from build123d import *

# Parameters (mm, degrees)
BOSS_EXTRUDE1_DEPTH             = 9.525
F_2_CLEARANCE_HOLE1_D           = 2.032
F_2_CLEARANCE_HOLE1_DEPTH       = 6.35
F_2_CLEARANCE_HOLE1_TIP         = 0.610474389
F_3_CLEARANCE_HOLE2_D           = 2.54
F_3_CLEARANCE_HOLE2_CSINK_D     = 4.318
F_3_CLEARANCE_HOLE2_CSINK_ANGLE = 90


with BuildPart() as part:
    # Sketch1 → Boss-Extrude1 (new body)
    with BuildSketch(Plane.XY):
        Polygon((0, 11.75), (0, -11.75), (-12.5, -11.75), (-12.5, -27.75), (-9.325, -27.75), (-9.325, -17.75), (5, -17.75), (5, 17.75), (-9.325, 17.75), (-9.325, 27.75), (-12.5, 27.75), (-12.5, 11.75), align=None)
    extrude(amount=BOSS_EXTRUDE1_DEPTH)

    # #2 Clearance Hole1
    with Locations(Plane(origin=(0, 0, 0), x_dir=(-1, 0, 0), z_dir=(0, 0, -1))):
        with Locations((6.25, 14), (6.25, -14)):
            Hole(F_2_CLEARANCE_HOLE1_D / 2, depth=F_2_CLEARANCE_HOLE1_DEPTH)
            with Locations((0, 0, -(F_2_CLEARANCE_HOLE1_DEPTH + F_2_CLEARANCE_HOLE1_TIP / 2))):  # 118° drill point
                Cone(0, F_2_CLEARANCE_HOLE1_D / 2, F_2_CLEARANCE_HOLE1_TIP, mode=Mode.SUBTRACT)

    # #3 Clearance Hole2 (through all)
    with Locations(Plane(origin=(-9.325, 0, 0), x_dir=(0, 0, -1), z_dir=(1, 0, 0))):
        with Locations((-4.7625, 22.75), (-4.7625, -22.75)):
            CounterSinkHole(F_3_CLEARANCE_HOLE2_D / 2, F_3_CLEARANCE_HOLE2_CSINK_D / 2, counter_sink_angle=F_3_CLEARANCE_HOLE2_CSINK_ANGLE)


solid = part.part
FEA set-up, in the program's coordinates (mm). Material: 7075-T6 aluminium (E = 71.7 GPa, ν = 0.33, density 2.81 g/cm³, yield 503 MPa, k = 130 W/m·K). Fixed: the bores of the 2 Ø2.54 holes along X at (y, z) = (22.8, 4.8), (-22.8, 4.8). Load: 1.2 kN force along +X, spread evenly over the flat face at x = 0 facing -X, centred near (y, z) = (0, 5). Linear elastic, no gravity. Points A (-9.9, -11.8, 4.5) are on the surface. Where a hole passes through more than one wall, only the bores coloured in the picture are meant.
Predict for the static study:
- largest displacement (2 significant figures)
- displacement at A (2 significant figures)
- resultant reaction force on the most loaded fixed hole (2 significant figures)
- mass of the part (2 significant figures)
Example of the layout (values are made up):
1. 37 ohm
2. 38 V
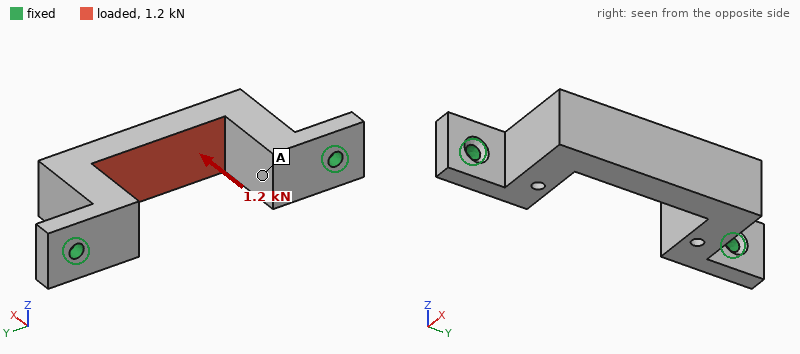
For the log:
1. 36 µm
2. 17 µm
3. 760 N
4. 10 g
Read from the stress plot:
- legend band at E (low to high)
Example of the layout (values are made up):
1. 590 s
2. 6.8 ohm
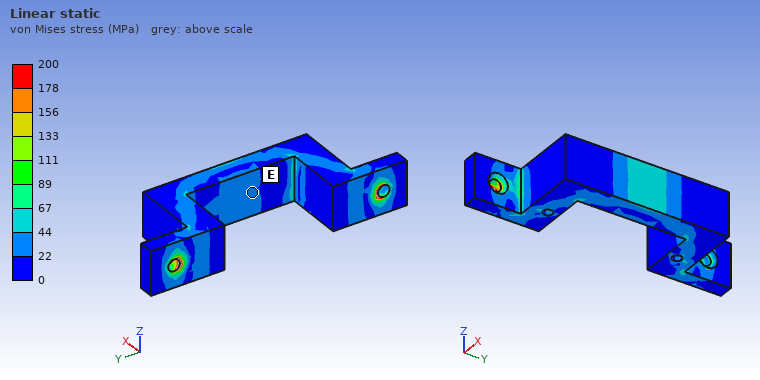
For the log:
1. 22 to 44 MPa
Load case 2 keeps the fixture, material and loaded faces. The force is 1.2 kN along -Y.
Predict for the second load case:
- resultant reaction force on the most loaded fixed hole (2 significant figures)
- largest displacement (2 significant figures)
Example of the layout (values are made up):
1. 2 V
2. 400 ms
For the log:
1. 660 N
2. 60 µm
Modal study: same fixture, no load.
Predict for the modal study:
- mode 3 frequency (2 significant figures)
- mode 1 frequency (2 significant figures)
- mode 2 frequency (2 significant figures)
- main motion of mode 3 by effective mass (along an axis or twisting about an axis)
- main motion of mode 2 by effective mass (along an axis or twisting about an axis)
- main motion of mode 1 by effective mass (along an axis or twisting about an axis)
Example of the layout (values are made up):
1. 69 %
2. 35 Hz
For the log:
1. 11 kHz
2. 3900 Hz
3. 9600 Hz
4. twisting about X
5. along Y
6. along Z
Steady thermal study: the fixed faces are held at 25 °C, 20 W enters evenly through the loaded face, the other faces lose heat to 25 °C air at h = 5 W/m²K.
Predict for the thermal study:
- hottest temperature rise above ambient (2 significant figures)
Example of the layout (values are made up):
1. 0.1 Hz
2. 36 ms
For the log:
1. 47 K
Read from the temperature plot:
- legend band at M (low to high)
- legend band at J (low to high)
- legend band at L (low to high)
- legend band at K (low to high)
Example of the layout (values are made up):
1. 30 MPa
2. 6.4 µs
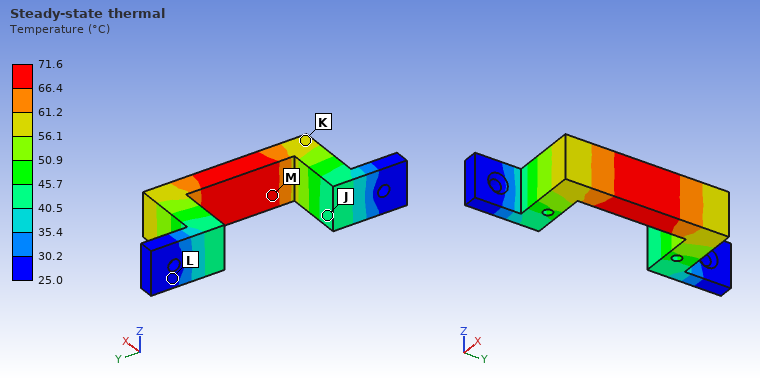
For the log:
1. 66.4 to 71.6 °C
2. 40.5 to 45.7 °C
3. 25.0 to 30.2 °C
4. 56.1 to 61.2 °C
